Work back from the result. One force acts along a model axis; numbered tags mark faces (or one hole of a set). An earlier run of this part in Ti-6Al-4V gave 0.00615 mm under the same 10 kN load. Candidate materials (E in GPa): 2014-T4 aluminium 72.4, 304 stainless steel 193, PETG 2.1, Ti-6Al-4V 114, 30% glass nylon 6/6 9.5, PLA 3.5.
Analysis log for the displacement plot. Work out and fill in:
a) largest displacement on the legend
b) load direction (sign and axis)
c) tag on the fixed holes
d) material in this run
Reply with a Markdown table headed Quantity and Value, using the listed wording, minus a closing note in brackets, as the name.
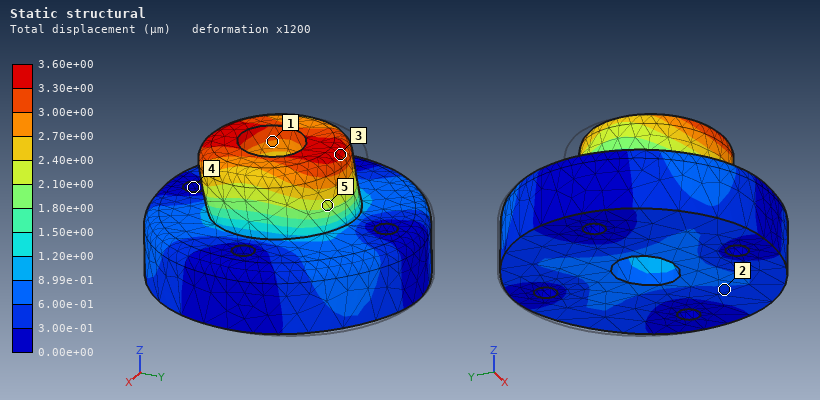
| Quantity | Value |
|---|---|
| largest displacement on the legend | 3.60e+00 µm |
| load direction | -Y |
| tag on the fixed holes | 4 |
| material in this run | 304 stainless steel |
